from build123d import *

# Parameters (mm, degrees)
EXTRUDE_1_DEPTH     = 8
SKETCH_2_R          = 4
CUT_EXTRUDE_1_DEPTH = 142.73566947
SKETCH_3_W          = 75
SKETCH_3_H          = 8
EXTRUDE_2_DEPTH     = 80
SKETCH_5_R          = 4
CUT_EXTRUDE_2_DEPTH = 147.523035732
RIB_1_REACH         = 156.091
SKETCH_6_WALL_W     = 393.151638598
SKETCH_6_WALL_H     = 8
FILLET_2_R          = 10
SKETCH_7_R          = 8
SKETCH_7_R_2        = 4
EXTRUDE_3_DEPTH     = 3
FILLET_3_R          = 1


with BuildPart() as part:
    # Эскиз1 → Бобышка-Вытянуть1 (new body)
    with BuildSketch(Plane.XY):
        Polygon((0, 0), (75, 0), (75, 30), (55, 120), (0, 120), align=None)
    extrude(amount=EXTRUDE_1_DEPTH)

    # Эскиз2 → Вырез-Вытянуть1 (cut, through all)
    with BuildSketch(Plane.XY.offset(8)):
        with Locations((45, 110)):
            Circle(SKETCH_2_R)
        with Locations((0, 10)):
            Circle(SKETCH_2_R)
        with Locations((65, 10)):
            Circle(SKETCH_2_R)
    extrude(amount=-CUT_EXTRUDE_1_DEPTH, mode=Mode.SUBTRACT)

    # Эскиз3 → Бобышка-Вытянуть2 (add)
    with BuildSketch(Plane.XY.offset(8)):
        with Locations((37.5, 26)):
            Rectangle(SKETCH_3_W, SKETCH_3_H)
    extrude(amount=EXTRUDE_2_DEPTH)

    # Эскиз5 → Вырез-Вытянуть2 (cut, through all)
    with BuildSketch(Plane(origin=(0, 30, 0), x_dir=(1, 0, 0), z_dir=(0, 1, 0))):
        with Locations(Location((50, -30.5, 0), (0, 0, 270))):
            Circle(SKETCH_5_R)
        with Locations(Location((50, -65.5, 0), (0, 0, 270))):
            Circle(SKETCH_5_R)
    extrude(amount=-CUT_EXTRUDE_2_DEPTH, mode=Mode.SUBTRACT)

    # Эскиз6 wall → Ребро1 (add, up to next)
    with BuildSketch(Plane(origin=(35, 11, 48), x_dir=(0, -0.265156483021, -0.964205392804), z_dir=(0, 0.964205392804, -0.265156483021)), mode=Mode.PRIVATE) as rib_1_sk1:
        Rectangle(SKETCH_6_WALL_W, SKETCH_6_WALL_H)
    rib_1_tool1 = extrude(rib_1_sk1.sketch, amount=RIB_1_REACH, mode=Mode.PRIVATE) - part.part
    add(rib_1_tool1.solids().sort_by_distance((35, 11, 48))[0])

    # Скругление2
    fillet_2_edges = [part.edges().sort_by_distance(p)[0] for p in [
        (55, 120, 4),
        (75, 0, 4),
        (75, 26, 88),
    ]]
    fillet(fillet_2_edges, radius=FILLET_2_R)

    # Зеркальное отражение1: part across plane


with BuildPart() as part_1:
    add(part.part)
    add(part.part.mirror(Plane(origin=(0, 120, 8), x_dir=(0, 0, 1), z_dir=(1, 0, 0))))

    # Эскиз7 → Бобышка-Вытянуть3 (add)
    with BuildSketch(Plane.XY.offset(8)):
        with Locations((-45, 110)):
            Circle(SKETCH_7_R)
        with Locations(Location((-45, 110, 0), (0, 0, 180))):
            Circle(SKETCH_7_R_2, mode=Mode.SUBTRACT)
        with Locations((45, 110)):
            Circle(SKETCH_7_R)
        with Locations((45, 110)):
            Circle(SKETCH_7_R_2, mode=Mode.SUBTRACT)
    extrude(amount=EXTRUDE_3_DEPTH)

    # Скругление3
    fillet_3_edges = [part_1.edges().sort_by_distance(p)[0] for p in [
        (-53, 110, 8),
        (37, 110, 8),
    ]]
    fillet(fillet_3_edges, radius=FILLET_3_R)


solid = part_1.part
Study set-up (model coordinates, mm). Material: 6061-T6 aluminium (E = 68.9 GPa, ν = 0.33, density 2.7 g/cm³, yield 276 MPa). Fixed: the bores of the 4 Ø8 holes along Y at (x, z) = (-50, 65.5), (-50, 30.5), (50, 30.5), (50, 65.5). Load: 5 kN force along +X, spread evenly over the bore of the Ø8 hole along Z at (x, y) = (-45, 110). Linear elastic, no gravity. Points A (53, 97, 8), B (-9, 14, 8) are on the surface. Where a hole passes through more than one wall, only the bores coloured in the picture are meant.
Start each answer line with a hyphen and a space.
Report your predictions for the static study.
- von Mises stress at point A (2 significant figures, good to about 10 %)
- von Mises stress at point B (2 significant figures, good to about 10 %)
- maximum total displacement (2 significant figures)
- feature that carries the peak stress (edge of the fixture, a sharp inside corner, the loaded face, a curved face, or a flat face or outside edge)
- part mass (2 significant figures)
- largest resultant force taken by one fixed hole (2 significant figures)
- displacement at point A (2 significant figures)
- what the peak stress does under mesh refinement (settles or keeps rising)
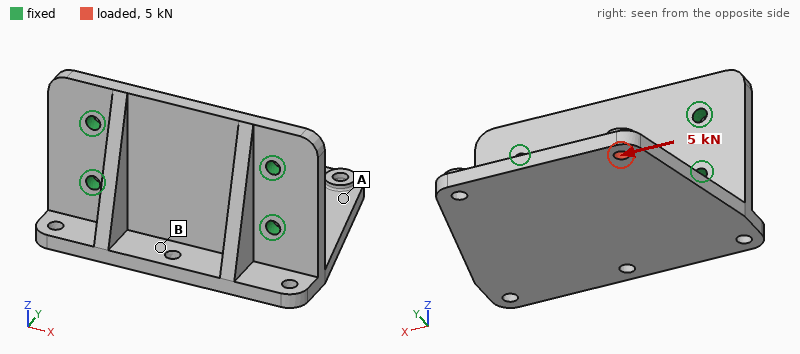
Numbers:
- 7.9 MPa
- 17 MPa
- 0.27 mm
- edge of the fixture
- 640 g
- 5.6 kN
- 0.20 mm
- keeps rising
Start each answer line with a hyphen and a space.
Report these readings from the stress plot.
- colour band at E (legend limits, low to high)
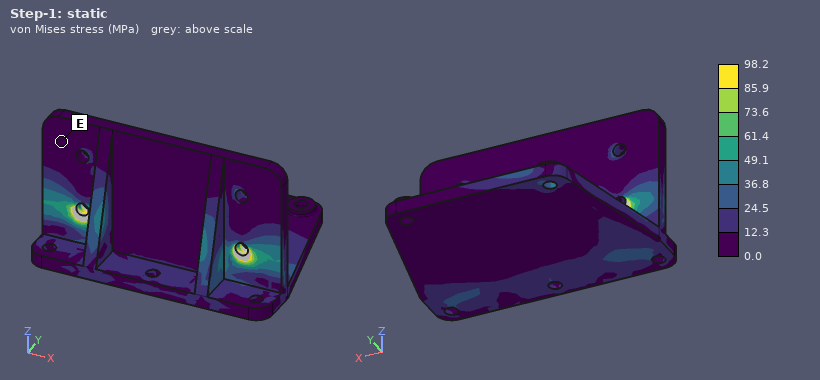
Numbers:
- 0.0 to 12.3 MPa
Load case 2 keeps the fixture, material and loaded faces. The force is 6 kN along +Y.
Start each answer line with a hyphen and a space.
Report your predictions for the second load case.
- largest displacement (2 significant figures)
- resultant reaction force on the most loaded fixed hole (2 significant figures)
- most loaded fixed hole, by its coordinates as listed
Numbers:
- 0.22 mm
- 7.6 kN
- (-50, 30.5)
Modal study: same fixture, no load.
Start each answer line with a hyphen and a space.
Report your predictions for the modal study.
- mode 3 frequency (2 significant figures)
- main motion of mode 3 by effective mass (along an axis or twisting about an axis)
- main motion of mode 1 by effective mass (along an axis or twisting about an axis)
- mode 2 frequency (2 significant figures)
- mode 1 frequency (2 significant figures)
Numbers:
- 2400 Hz
- along X
- along Z
- 1500 Hz
- 700 Hz
